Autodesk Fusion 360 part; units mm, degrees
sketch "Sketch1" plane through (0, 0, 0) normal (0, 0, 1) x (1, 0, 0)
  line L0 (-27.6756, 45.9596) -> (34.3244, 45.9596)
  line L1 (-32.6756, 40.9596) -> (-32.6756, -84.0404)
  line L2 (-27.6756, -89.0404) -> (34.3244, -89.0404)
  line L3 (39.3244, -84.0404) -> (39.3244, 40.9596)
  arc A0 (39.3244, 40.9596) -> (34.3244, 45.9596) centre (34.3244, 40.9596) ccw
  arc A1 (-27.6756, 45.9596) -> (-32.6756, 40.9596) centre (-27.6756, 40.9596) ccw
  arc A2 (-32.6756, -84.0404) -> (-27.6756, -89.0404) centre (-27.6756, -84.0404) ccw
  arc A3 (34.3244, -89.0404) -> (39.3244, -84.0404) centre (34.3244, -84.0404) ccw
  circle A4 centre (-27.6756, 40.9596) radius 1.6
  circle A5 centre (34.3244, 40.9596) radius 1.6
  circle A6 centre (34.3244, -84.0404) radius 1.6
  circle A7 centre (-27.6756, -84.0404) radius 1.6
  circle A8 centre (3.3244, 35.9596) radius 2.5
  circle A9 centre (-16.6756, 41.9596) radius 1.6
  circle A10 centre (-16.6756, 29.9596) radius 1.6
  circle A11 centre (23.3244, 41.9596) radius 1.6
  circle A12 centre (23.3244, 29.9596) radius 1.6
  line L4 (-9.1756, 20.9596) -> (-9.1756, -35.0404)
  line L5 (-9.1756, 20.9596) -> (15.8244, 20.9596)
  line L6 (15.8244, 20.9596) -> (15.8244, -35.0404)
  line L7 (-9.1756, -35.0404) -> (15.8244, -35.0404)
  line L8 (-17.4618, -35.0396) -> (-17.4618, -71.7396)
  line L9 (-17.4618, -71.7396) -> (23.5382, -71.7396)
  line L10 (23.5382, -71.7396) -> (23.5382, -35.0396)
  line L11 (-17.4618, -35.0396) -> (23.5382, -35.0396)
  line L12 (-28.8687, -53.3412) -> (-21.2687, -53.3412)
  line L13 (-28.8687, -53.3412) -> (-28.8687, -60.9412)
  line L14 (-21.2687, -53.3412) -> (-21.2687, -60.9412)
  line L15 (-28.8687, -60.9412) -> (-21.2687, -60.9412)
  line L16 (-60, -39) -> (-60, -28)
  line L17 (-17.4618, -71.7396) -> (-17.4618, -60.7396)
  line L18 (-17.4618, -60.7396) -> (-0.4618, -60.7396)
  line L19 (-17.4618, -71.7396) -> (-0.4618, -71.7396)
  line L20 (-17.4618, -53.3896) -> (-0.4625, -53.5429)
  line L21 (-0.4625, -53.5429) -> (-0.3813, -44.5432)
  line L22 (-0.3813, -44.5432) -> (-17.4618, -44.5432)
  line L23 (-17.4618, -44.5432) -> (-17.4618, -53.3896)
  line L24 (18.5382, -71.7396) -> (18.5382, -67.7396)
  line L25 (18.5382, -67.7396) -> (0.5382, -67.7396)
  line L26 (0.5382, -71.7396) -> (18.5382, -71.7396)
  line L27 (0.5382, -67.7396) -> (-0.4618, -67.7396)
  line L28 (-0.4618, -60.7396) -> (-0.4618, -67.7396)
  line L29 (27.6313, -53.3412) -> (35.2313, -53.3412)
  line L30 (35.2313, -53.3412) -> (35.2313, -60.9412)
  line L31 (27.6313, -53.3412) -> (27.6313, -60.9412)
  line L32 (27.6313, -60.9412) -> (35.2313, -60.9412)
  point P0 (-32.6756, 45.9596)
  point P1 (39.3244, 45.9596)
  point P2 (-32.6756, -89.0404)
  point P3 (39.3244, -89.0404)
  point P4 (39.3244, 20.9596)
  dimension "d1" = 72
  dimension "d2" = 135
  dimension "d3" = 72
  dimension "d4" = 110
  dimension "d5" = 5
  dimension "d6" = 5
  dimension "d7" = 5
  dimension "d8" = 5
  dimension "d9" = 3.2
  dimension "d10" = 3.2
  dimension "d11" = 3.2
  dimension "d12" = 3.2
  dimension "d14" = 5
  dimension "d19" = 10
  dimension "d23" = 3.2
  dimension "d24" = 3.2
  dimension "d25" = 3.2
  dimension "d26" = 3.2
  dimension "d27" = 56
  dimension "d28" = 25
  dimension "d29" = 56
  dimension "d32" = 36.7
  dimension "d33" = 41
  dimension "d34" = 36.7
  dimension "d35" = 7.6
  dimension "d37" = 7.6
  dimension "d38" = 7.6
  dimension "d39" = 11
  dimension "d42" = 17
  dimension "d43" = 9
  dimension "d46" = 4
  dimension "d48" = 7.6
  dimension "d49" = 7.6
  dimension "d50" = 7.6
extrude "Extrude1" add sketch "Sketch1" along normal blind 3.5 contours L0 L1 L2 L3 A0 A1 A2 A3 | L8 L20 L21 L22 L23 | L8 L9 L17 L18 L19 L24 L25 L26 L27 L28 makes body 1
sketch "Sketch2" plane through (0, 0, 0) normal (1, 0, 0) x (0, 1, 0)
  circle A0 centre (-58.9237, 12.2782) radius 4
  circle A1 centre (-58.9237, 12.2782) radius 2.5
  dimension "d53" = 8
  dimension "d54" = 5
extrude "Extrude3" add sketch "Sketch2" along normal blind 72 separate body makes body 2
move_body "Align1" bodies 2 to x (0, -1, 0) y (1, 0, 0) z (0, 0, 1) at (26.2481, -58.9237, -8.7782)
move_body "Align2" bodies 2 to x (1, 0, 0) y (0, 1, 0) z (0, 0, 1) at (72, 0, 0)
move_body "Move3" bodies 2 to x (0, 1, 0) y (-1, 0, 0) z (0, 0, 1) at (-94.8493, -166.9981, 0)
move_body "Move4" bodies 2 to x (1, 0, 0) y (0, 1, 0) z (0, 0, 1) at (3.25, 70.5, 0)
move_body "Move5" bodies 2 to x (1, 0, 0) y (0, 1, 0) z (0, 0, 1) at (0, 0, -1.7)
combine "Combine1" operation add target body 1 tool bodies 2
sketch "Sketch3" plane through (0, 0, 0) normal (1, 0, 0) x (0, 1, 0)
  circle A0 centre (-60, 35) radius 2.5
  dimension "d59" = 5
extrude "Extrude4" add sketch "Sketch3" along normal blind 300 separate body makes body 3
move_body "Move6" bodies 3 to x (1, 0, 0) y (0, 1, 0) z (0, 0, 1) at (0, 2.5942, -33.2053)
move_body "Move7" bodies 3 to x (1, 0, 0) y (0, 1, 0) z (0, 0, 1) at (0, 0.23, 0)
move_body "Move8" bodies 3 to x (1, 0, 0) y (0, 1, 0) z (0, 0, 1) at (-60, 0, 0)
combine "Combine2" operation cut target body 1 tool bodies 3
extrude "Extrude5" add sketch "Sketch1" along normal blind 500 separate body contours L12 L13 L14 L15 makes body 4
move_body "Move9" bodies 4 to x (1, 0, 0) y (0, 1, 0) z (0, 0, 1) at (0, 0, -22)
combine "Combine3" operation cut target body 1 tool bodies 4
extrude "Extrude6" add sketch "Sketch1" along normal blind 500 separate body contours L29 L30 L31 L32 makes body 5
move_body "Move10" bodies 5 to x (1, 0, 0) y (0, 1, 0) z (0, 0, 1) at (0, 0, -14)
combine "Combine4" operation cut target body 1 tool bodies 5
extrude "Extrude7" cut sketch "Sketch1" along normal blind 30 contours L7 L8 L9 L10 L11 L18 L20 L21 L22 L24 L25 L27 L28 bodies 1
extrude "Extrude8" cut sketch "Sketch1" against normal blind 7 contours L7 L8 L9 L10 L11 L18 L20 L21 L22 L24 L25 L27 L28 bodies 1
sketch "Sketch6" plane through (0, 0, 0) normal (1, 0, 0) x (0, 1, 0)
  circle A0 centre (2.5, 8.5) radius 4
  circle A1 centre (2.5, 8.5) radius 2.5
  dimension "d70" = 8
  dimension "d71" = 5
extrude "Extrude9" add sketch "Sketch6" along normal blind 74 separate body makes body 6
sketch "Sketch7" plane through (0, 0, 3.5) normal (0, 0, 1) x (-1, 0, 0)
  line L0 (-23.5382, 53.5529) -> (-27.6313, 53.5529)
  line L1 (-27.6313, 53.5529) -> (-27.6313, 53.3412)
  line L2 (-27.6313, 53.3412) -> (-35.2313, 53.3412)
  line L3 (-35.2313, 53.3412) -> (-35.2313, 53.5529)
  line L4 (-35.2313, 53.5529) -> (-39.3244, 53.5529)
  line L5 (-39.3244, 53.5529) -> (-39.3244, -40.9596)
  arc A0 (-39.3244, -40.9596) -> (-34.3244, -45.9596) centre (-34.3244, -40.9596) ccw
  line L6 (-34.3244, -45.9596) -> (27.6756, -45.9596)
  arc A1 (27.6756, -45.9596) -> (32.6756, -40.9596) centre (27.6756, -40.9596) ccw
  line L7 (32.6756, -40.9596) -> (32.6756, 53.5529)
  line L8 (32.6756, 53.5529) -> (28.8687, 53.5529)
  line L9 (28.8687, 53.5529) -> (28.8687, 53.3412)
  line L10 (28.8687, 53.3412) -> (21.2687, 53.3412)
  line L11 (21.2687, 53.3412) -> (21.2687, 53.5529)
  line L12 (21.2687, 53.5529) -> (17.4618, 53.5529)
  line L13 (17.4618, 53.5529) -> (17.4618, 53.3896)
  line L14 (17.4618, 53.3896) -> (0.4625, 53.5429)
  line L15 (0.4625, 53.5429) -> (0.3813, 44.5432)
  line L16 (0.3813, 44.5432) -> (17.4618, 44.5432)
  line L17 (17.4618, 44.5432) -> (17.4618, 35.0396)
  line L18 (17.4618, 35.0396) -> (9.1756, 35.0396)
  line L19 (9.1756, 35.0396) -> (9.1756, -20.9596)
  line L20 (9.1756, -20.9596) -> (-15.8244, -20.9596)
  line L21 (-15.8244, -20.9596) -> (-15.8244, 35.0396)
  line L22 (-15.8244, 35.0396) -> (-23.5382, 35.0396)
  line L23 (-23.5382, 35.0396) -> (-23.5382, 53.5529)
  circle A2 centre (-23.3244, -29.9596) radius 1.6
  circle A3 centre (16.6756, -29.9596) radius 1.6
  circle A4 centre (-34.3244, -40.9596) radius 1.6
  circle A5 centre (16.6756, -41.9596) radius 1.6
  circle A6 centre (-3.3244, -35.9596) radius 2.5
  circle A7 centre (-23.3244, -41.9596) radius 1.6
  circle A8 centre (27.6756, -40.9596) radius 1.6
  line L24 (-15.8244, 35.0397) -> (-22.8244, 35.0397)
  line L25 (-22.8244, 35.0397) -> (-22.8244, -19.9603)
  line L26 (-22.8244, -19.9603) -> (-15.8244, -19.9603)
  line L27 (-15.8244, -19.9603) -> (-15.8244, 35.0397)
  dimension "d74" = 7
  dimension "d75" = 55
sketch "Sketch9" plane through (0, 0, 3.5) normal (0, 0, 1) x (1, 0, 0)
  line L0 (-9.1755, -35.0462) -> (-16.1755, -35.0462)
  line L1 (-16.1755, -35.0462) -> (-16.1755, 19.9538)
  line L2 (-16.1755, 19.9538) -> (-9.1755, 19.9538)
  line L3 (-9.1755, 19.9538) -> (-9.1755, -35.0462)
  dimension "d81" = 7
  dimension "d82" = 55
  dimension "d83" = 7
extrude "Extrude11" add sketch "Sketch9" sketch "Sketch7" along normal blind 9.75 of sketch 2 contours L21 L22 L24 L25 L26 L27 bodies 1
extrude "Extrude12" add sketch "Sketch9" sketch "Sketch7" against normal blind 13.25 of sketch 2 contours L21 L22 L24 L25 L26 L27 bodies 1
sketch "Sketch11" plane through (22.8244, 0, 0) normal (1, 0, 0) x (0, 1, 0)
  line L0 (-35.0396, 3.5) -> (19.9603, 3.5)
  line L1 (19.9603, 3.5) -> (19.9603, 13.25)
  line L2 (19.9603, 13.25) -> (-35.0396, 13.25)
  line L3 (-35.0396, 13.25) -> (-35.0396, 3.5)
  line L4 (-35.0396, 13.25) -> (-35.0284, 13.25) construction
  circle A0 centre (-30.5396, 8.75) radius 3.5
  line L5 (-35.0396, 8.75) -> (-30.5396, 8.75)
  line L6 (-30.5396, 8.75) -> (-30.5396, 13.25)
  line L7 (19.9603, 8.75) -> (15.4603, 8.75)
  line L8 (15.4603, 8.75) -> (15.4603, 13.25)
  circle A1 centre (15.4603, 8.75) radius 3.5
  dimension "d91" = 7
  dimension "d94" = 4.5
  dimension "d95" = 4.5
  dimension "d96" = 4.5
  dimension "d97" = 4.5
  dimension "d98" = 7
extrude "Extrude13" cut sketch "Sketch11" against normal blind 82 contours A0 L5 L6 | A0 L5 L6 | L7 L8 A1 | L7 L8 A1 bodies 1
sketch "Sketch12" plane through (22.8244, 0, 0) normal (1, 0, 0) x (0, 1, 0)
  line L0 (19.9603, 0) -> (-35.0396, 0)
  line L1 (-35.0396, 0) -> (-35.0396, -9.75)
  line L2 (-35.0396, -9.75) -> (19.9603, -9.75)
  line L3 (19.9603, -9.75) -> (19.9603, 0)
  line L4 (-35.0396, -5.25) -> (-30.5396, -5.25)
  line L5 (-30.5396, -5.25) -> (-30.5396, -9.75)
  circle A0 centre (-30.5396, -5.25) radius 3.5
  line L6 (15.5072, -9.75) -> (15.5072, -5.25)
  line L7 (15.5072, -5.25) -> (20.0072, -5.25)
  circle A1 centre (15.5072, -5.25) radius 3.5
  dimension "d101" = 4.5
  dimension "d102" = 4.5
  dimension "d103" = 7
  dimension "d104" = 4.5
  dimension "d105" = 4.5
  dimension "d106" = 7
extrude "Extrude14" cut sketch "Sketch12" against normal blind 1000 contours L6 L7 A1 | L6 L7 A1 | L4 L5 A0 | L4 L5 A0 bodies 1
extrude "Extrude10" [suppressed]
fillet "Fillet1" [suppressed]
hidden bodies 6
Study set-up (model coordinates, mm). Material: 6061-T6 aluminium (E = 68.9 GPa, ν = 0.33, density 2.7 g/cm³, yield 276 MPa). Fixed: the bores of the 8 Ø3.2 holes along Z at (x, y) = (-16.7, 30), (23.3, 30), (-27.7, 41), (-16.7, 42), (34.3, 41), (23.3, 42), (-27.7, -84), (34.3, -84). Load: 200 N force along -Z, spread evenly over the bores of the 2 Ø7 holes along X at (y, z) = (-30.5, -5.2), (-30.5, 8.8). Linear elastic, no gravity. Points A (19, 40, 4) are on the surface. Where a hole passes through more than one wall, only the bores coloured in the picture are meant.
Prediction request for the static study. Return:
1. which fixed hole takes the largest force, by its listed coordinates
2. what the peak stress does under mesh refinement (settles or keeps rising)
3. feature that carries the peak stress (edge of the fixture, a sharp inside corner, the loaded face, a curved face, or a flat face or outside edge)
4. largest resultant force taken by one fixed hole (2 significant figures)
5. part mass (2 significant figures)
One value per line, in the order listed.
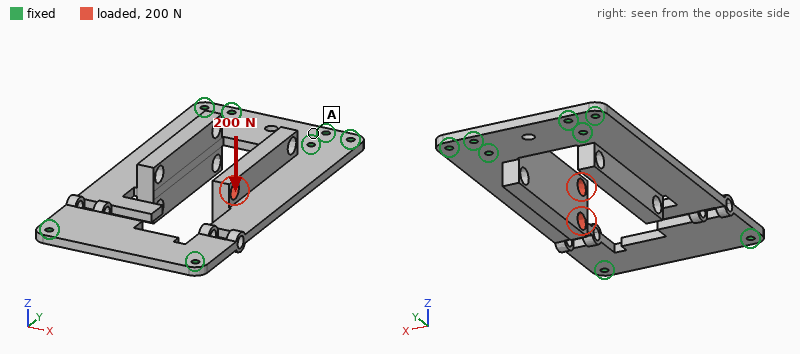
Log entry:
(23.3, 30)
keeps rising
a sharp inside corner
210 N
100 g
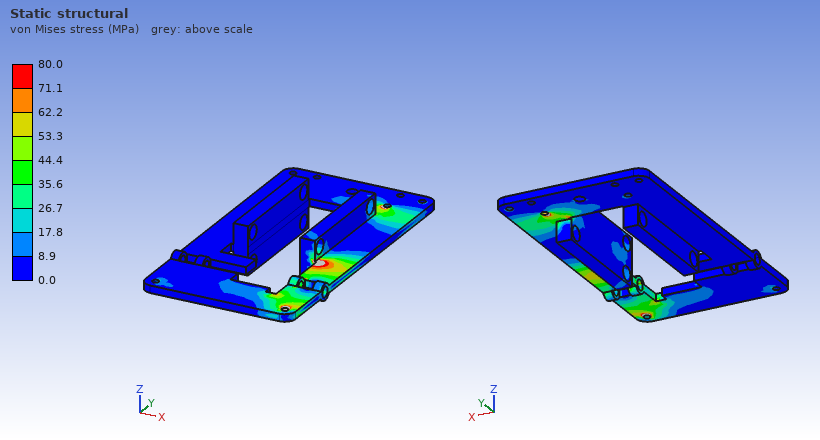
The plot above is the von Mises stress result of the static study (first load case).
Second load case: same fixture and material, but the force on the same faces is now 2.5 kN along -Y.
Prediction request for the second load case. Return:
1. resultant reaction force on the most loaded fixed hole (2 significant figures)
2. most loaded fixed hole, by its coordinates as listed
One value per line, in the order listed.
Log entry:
1.4 kN
(23.3, 30)
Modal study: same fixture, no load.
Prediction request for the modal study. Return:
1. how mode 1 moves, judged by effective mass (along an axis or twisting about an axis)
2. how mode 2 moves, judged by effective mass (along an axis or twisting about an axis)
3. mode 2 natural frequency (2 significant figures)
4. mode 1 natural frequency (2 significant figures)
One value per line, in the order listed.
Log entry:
along Z
twisting about Y
1100 Hz
1100 Hz
